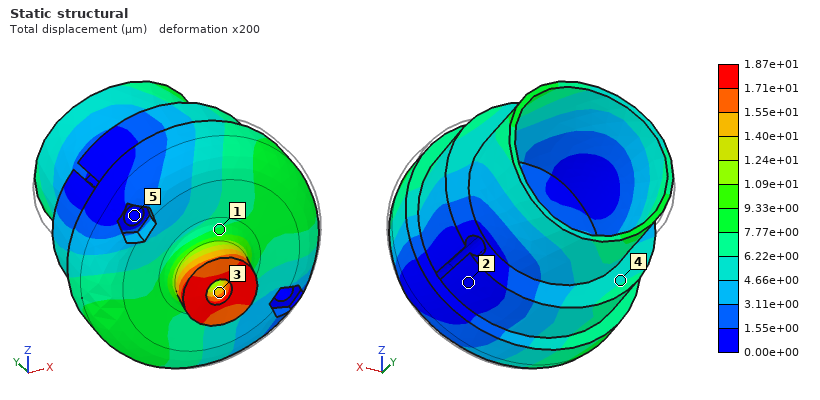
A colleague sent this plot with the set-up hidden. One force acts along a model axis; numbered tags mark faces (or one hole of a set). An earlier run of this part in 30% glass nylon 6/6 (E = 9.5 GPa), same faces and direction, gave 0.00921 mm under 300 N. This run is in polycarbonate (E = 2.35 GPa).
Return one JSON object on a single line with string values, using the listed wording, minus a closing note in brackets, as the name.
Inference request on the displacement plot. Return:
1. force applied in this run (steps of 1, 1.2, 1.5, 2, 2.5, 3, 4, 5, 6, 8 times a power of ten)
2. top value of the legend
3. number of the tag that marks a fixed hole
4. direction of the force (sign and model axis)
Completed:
{"force applied in this run": "150 N", "top value of the legend": "1.87e+01 µm", "number of the tag that marks a fixed hole": "5", "direction of the force": "-X"}
